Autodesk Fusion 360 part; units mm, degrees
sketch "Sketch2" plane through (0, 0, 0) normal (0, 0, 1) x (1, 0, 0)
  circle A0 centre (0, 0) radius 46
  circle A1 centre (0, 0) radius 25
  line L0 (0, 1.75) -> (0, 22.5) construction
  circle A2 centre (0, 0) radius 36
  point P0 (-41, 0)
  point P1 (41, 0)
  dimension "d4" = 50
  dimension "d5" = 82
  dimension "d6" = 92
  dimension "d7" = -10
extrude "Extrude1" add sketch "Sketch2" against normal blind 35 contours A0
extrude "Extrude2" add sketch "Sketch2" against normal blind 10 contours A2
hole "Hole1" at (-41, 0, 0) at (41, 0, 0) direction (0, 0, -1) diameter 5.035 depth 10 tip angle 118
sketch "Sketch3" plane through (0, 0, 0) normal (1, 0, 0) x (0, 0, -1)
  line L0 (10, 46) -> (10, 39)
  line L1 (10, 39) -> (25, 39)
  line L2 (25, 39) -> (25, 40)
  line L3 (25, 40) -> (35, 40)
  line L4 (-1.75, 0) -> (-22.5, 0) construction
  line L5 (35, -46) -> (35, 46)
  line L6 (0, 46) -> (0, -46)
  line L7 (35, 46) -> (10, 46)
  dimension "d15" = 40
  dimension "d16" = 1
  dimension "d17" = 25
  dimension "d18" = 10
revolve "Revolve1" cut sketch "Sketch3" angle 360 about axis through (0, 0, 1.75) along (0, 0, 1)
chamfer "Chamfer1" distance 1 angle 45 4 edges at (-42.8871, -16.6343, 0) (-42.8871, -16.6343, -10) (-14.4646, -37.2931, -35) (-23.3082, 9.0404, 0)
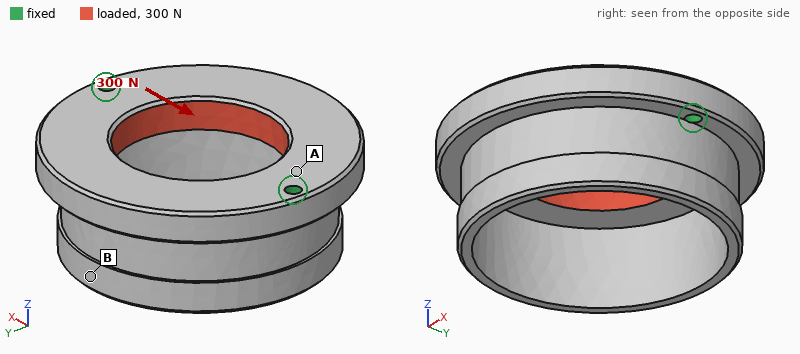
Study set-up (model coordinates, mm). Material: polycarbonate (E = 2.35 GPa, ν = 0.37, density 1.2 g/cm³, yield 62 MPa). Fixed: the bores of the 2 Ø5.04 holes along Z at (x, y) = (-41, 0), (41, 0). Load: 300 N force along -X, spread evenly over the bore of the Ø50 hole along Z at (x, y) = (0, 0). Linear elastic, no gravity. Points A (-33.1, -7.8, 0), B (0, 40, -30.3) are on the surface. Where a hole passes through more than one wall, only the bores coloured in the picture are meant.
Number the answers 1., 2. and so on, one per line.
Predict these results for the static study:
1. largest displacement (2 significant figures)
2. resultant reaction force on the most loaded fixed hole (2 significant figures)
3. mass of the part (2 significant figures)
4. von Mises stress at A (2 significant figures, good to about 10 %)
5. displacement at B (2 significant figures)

1. 17 µm
2. 150 N
3. 79 g
4. 0.78 MPa
5. 12 µm
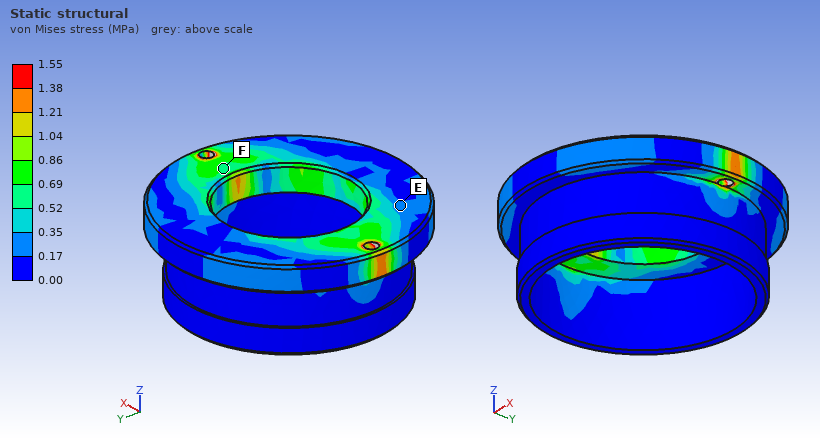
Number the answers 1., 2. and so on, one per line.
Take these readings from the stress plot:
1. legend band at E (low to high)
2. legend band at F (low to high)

1. 0.17 to 0.35 MPa
2. 0.52 to 0.69 MPa
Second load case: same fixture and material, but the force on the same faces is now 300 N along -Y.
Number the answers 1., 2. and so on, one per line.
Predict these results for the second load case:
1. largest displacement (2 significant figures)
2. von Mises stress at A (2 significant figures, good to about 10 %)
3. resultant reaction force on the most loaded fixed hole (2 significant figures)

1. 12 µm
2. 0.52 MPa
3. 150 N
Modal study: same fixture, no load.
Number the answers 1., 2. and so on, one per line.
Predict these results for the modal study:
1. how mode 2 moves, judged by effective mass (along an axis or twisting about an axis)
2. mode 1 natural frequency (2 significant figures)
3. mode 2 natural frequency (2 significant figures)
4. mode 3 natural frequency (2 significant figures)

1. along Z
2. 690 Hz
3. 870 Hz
4. 1400 Hz
